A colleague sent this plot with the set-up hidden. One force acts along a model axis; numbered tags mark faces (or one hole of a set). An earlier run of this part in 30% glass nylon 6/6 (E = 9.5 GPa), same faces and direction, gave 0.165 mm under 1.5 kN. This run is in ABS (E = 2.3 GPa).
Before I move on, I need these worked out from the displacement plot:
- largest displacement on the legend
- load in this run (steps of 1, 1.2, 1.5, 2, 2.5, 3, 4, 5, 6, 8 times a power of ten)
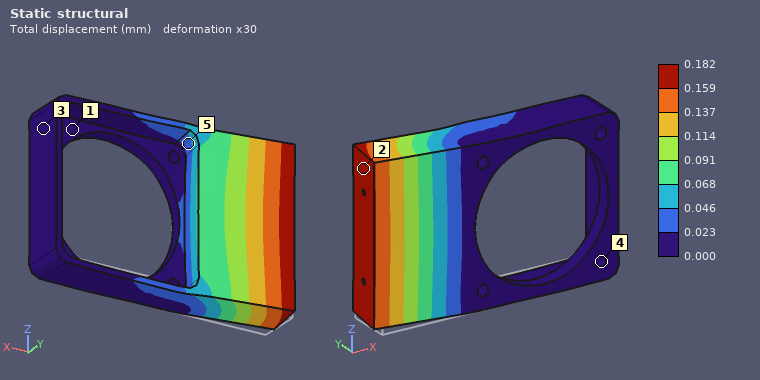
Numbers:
0.182 mm
400 N
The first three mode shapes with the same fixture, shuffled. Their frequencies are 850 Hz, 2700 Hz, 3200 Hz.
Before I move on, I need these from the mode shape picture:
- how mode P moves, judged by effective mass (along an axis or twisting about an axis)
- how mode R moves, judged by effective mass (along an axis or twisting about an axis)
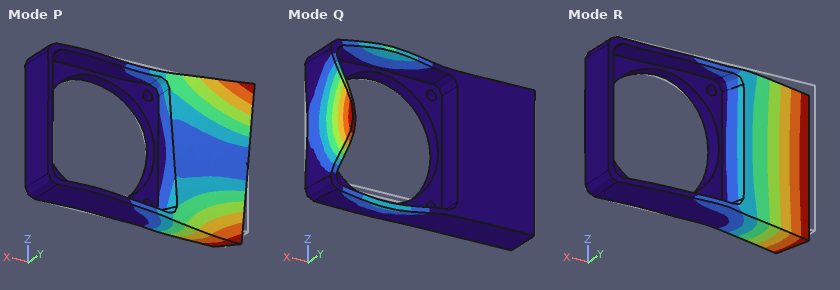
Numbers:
twisting about X
along Y
